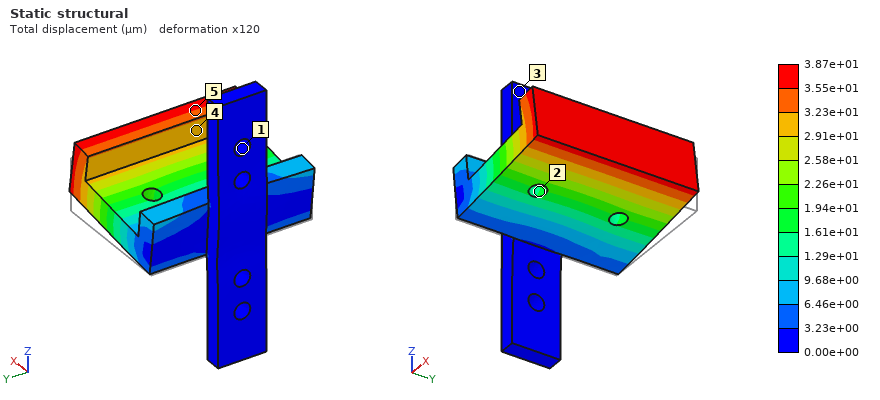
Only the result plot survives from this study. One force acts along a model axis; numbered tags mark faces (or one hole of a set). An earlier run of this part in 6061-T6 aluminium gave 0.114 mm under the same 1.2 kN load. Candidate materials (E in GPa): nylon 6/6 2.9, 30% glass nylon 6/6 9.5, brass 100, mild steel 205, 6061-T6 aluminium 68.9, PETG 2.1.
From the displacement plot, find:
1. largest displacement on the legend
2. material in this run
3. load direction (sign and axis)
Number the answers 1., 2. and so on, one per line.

1. 3.87e+01 µm
2. mild steel
3. +Z
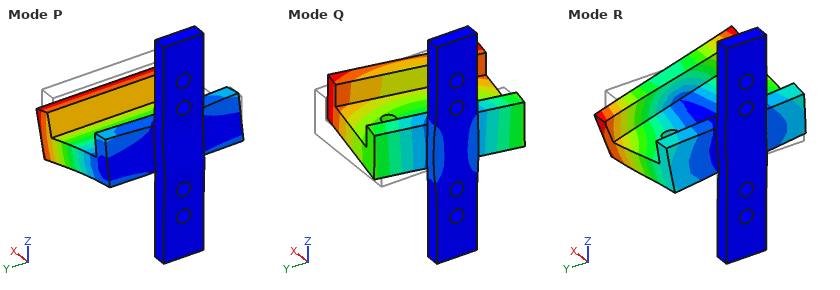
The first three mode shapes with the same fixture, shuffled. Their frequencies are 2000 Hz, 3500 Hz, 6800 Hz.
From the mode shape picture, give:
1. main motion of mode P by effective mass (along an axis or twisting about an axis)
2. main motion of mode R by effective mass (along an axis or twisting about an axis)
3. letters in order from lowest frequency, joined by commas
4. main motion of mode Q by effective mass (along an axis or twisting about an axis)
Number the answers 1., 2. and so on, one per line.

1. along Z
2. twisting about X
3. Q, P, R
4. along Y
